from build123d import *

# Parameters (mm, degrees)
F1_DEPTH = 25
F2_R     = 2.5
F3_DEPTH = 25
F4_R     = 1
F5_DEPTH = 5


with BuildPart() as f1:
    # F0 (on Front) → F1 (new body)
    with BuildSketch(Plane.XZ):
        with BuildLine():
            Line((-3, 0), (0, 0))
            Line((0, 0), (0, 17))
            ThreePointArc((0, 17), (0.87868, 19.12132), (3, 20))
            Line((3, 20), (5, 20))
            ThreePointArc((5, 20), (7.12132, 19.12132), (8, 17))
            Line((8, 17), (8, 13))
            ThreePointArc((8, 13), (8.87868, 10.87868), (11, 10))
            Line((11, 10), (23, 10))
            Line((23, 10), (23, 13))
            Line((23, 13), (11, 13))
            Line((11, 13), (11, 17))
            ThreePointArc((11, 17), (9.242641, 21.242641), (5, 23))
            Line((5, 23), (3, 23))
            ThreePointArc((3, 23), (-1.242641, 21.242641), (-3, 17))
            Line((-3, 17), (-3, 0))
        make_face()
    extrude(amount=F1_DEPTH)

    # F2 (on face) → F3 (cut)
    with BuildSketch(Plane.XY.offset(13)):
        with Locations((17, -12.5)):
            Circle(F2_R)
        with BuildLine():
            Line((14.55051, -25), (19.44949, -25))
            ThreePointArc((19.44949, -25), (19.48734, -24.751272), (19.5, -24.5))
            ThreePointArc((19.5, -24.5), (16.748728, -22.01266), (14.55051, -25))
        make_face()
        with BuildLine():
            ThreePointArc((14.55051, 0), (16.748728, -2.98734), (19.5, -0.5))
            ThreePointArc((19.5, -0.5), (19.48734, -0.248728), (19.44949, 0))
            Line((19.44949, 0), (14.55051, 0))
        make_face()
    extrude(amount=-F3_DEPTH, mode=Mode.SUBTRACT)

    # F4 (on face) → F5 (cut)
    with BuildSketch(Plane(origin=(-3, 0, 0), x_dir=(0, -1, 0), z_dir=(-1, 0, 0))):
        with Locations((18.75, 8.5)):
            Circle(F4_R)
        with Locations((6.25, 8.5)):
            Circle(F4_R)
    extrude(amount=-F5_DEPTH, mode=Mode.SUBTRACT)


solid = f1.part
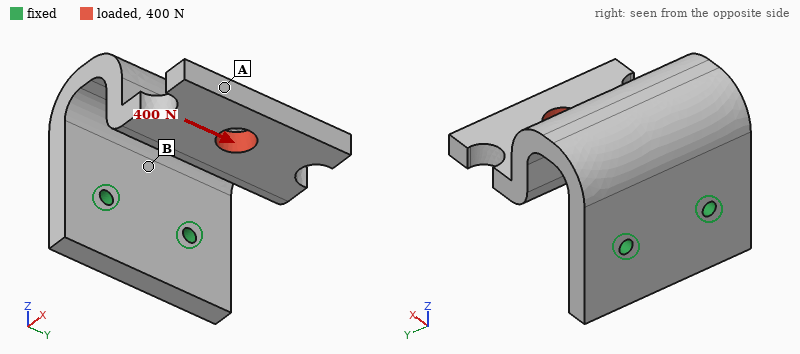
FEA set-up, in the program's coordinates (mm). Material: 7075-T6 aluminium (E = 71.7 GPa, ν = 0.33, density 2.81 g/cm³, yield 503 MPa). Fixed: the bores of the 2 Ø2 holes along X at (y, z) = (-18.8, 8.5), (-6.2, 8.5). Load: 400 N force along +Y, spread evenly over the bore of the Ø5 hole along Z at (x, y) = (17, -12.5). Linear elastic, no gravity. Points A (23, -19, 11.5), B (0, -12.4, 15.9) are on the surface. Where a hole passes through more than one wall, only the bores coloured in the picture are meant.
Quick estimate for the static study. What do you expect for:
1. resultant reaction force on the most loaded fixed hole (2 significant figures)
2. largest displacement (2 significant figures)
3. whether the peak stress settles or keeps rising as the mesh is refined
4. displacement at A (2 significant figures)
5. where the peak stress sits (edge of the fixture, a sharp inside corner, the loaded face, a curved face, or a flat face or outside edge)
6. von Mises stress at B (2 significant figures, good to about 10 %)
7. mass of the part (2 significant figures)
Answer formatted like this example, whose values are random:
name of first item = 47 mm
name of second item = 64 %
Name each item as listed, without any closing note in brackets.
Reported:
resultant reaction force on the most loaded fixed hole = 510 N
largest displacement = 0.33 mm
whether the peak stress settles or keeps rising as the mesh is refined = keeps rising
displacement at A = 0.30 mm
where the peak stress sits = edge of the fixture
von Mises stress at B = 130 MPa
mass of the part = 10 g
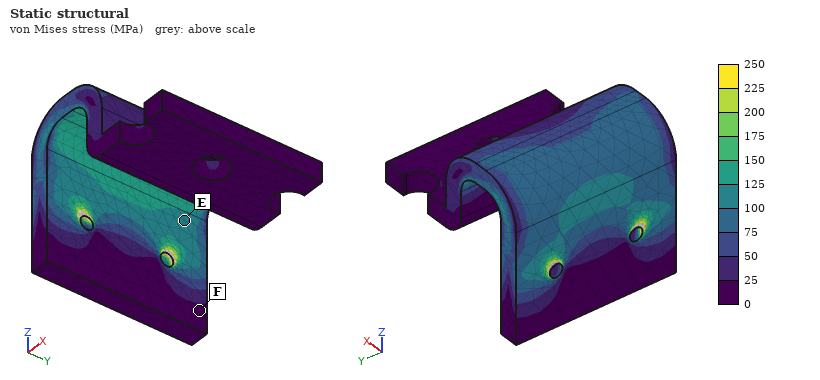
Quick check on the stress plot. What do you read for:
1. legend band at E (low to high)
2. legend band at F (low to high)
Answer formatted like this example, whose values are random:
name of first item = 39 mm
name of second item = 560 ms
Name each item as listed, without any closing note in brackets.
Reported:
legend band at E = 100 to 125 MPa
legend band at F = 0 to 25 MPa
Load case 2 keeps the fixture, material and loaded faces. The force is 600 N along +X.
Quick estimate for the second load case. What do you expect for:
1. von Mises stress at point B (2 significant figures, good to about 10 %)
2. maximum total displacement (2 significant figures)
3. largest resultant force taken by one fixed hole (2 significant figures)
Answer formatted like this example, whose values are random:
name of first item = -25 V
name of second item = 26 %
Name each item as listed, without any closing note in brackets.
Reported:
von Mises stress at point B = 64 MPa
maximum total displacement = 0.47 mm
largest resultant force taken by one fixed hole = 300 N
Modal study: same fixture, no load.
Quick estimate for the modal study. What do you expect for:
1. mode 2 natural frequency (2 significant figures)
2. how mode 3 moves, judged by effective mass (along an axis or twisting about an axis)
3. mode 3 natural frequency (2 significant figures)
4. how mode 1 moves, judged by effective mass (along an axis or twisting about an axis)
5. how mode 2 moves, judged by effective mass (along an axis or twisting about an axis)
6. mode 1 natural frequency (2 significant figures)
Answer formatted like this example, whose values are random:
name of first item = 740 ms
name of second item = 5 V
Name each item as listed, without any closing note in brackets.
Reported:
mode 2 natural frequency = 3400 Hz
how mode 3 moves, judged by effective mass = along X
mode 3 natural frequency = 5300 Hz
how mode 1 moves, judged by effective mass = along Z
how mode 2 moves, judged by effective mass = along Y
mode 1 natural frequency = 2200 Hz
